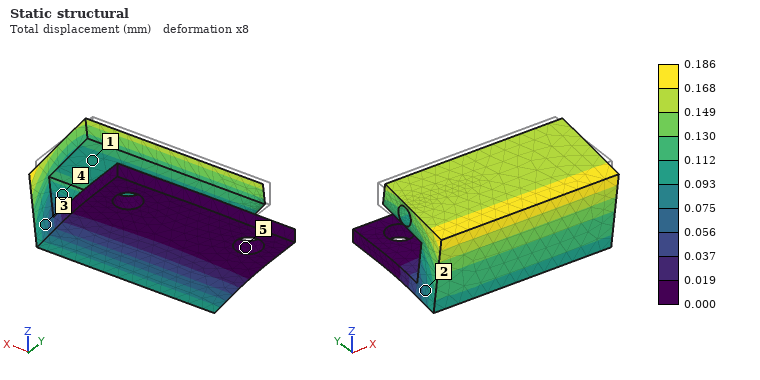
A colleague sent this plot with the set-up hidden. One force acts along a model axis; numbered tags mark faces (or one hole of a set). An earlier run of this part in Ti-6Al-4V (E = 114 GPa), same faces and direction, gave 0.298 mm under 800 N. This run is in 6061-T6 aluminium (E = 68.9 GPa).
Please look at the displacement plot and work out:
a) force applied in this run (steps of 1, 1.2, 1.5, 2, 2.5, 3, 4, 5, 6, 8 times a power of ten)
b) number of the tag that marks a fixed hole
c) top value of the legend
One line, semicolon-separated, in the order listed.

300 N; 5; 0.186 mm
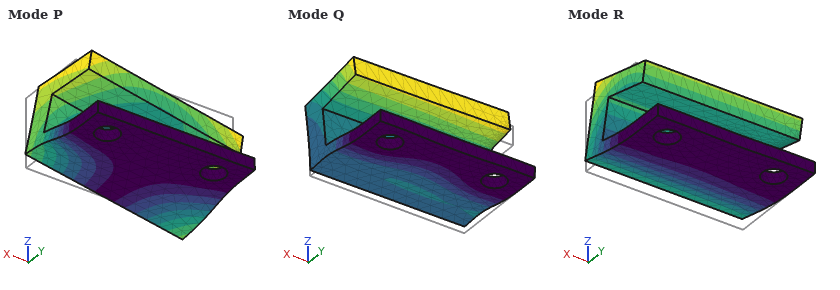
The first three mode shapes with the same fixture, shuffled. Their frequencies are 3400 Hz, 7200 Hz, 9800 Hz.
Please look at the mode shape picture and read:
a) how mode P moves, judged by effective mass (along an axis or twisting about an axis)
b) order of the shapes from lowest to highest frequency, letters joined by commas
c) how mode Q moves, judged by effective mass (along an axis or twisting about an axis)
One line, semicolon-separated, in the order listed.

along X; R, P, Q; along Z
